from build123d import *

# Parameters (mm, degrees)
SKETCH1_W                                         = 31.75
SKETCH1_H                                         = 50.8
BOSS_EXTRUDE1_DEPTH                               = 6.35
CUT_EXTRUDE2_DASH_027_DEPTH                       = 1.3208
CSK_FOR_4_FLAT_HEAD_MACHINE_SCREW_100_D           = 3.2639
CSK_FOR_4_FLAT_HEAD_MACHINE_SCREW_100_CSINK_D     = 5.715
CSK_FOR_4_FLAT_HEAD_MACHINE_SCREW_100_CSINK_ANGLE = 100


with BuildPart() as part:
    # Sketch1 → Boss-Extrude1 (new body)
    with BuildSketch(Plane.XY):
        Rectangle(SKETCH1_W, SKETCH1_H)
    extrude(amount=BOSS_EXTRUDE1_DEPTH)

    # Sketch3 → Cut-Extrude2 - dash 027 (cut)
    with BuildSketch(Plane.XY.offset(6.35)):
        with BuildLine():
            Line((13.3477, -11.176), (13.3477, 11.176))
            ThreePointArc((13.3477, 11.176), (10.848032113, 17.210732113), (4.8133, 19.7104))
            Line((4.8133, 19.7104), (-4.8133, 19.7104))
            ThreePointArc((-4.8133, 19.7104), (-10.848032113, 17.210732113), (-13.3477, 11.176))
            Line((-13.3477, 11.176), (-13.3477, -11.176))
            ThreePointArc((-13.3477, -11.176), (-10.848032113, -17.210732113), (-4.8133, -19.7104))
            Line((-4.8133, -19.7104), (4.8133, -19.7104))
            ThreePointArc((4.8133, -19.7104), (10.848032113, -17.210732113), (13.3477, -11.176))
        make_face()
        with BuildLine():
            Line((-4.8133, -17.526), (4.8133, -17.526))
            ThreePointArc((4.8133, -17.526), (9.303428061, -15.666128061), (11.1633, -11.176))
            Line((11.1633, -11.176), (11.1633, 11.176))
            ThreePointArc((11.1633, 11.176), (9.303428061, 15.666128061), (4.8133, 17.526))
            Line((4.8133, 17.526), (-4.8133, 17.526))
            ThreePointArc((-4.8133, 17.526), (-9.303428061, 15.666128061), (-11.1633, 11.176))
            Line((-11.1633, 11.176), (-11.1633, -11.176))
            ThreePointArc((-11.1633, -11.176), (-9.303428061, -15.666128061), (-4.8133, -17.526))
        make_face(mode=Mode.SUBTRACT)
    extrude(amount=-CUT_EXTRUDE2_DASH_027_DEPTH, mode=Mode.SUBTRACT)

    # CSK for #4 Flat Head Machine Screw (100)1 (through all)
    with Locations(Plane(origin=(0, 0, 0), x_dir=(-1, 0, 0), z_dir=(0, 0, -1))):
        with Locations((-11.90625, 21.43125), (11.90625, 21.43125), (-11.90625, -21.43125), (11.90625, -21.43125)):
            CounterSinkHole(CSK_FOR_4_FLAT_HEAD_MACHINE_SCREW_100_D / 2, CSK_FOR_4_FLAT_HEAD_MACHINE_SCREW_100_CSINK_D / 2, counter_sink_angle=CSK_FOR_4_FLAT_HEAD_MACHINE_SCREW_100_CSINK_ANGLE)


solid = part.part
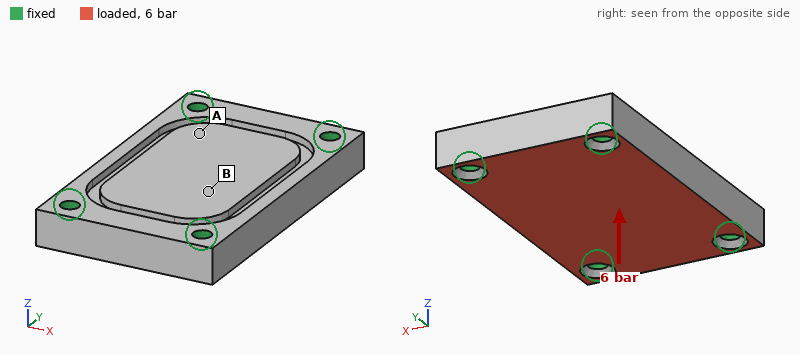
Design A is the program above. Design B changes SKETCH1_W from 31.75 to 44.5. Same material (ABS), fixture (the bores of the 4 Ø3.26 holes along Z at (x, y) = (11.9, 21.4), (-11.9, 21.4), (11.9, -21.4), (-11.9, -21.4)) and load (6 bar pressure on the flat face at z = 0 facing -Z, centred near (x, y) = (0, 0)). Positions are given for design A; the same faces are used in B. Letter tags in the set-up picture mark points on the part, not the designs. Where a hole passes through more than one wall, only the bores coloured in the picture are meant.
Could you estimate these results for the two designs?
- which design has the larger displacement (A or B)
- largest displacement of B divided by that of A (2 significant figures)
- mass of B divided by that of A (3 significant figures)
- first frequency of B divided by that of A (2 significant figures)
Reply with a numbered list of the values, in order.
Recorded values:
1. B
2. 1.2
3. 1.42
4. 0.95
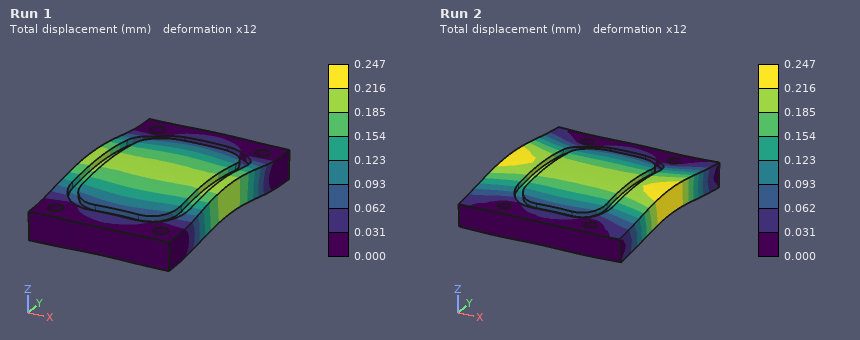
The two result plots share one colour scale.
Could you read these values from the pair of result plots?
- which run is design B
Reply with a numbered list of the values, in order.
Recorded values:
1. Run 2
